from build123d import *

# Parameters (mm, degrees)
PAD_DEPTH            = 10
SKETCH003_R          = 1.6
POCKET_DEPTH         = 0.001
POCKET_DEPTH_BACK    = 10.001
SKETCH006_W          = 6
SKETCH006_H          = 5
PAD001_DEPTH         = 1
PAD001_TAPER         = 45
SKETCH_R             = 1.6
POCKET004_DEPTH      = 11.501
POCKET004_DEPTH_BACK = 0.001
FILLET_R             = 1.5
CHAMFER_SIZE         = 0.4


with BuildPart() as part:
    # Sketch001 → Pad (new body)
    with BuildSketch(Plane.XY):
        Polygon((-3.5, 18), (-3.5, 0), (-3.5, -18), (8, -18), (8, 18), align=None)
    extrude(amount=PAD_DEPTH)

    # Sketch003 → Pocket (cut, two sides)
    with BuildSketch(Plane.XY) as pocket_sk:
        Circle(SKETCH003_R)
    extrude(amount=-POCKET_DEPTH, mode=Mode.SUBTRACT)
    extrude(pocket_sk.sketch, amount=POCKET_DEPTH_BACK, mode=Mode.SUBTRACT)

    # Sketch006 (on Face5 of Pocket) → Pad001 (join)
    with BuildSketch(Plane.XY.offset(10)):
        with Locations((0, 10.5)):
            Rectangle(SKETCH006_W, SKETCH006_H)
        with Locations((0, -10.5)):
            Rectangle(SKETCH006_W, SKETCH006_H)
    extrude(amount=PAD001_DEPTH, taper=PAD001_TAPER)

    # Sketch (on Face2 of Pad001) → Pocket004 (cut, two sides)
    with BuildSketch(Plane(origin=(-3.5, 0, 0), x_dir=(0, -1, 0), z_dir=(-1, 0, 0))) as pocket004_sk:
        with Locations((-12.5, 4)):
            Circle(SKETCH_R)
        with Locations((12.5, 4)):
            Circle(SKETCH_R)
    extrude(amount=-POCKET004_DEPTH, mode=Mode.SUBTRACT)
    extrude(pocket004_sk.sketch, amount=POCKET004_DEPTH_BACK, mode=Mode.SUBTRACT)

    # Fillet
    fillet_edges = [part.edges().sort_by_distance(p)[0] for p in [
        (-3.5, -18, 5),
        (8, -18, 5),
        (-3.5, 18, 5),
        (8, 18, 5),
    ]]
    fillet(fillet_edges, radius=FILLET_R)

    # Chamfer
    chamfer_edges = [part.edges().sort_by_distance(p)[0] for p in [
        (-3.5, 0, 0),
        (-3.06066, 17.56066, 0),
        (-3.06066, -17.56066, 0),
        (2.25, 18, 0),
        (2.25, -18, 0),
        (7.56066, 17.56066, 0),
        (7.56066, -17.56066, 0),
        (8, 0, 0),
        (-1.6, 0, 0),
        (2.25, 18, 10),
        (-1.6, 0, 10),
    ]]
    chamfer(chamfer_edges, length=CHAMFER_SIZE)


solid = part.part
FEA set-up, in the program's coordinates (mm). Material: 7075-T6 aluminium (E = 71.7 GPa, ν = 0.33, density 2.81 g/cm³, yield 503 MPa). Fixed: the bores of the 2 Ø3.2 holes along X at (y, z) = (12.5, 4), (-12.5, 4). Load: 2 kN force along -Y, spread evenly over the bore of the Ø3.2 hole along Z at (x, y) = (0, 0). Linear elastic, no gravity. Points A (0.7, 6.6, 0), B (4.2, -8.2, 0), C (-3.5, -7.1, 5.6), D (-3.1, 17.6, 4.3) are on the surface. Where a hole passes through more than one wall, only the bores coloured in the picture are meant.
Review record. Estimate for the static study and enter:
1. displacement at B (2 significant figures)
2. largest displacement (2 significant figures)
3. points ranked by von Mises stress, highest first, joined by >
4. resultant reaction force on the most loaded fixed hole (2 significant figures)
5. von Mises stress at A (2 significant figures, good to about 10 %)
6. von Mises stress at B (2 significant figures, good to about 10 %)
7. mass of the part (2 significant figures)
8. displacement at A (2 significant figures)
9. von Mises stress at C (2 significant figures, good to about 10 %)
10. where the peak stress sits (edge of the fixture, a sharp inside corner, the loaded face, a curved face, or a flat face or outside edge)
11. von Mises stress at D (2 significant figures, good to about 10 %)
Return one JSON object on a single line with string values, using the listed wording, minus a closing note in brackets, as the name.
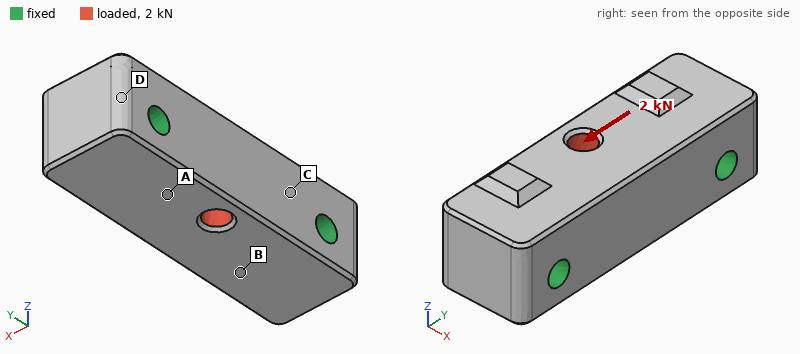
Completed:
{"displacement at B": "0.55 µm", "largest displacement": "2.6 µm", "points ranked by von Mises stress, highest first, joined by >": "C > A > B > D", "resultant reaction force on the most loaded fixed hole": "1.0 kN", "von Mises stress at A": "12 MPa", "von Mises stress at B": "7.2 MPa", "mass of the part": "11 g", "displacement at A": "0.90 µm", "von Mises stress at C": "15 MPa", "where the peak stress sits": "the loaded face", "von Mises stress at D": "3.3 MPa"}
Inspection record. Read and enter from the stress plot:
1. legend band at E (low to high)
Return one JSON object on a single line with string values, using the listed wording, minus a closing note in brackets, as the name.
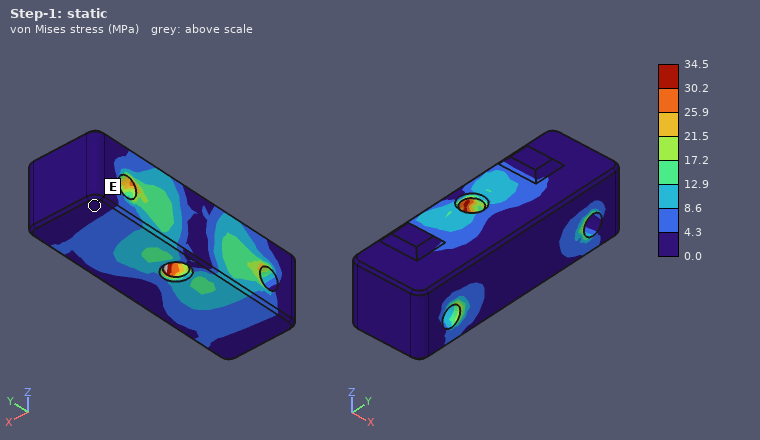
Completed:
{"legend band at E": "0.0 to 4.3 MPa"}
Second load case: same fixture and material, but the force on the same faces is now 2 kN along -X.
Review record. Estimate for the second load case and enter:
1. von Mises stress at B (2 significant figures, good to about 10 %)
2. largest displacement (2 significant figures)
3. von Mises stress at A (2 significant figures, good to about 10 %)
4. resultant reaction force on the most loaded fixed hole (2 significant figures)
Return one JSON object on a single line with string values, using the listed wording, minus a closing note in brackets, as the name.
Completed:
{"von Mises stress at B": "20 MPa", "largest displacement": "7.3 µm", "von Mises stress at A": "22 MPa", "resultant reaction force on the most loaded fixed hole": "1.0 kN"}
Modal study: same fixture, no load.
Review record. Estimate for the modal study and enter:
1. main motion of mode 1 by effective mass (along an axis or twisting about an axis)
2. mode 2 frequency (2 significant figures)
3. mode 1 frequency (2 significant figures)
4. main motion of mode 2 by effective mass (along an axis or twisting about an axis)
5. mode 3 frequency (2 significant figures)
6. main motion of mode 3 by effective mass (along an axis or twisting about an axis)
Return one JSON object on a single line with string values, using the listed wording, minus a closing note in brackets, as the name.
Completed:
{"main motion of mode 1 by effective mass": "along Z", "mode 2 frequency": "51 kHz", "mode 1 frequency": "42 kHz", "main motion of mode 2 by effective mass": "along X", "mode 3 frequency": "60 kHz", "main motion of mode 3 by effective mass": "twisting about Y"}
